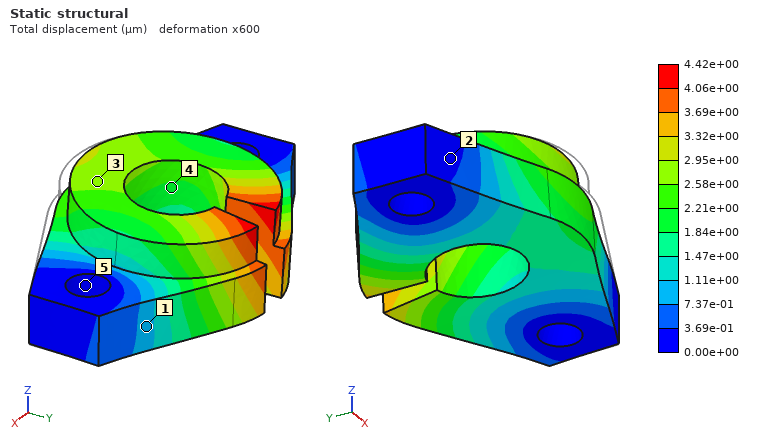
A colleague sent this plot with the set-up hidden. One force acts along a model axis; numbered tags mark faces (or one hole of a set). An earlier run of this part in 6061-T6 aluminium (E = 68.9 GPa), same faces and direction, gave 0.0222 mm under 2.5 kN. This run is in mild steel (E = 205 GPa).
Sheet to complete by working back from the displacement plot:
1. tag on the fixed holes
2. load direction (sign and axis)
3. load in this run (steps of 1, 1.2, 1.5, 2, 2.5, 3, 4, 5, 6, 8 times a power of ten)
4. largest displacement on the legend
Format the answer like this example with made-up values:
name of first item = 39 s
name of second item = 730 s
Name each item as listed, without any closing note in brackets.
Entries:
tag on the fixed holes = 5
load direction = +Y
load in this run = 1.5 kN
largest displacement on the legend = 4.42e+00 µm
